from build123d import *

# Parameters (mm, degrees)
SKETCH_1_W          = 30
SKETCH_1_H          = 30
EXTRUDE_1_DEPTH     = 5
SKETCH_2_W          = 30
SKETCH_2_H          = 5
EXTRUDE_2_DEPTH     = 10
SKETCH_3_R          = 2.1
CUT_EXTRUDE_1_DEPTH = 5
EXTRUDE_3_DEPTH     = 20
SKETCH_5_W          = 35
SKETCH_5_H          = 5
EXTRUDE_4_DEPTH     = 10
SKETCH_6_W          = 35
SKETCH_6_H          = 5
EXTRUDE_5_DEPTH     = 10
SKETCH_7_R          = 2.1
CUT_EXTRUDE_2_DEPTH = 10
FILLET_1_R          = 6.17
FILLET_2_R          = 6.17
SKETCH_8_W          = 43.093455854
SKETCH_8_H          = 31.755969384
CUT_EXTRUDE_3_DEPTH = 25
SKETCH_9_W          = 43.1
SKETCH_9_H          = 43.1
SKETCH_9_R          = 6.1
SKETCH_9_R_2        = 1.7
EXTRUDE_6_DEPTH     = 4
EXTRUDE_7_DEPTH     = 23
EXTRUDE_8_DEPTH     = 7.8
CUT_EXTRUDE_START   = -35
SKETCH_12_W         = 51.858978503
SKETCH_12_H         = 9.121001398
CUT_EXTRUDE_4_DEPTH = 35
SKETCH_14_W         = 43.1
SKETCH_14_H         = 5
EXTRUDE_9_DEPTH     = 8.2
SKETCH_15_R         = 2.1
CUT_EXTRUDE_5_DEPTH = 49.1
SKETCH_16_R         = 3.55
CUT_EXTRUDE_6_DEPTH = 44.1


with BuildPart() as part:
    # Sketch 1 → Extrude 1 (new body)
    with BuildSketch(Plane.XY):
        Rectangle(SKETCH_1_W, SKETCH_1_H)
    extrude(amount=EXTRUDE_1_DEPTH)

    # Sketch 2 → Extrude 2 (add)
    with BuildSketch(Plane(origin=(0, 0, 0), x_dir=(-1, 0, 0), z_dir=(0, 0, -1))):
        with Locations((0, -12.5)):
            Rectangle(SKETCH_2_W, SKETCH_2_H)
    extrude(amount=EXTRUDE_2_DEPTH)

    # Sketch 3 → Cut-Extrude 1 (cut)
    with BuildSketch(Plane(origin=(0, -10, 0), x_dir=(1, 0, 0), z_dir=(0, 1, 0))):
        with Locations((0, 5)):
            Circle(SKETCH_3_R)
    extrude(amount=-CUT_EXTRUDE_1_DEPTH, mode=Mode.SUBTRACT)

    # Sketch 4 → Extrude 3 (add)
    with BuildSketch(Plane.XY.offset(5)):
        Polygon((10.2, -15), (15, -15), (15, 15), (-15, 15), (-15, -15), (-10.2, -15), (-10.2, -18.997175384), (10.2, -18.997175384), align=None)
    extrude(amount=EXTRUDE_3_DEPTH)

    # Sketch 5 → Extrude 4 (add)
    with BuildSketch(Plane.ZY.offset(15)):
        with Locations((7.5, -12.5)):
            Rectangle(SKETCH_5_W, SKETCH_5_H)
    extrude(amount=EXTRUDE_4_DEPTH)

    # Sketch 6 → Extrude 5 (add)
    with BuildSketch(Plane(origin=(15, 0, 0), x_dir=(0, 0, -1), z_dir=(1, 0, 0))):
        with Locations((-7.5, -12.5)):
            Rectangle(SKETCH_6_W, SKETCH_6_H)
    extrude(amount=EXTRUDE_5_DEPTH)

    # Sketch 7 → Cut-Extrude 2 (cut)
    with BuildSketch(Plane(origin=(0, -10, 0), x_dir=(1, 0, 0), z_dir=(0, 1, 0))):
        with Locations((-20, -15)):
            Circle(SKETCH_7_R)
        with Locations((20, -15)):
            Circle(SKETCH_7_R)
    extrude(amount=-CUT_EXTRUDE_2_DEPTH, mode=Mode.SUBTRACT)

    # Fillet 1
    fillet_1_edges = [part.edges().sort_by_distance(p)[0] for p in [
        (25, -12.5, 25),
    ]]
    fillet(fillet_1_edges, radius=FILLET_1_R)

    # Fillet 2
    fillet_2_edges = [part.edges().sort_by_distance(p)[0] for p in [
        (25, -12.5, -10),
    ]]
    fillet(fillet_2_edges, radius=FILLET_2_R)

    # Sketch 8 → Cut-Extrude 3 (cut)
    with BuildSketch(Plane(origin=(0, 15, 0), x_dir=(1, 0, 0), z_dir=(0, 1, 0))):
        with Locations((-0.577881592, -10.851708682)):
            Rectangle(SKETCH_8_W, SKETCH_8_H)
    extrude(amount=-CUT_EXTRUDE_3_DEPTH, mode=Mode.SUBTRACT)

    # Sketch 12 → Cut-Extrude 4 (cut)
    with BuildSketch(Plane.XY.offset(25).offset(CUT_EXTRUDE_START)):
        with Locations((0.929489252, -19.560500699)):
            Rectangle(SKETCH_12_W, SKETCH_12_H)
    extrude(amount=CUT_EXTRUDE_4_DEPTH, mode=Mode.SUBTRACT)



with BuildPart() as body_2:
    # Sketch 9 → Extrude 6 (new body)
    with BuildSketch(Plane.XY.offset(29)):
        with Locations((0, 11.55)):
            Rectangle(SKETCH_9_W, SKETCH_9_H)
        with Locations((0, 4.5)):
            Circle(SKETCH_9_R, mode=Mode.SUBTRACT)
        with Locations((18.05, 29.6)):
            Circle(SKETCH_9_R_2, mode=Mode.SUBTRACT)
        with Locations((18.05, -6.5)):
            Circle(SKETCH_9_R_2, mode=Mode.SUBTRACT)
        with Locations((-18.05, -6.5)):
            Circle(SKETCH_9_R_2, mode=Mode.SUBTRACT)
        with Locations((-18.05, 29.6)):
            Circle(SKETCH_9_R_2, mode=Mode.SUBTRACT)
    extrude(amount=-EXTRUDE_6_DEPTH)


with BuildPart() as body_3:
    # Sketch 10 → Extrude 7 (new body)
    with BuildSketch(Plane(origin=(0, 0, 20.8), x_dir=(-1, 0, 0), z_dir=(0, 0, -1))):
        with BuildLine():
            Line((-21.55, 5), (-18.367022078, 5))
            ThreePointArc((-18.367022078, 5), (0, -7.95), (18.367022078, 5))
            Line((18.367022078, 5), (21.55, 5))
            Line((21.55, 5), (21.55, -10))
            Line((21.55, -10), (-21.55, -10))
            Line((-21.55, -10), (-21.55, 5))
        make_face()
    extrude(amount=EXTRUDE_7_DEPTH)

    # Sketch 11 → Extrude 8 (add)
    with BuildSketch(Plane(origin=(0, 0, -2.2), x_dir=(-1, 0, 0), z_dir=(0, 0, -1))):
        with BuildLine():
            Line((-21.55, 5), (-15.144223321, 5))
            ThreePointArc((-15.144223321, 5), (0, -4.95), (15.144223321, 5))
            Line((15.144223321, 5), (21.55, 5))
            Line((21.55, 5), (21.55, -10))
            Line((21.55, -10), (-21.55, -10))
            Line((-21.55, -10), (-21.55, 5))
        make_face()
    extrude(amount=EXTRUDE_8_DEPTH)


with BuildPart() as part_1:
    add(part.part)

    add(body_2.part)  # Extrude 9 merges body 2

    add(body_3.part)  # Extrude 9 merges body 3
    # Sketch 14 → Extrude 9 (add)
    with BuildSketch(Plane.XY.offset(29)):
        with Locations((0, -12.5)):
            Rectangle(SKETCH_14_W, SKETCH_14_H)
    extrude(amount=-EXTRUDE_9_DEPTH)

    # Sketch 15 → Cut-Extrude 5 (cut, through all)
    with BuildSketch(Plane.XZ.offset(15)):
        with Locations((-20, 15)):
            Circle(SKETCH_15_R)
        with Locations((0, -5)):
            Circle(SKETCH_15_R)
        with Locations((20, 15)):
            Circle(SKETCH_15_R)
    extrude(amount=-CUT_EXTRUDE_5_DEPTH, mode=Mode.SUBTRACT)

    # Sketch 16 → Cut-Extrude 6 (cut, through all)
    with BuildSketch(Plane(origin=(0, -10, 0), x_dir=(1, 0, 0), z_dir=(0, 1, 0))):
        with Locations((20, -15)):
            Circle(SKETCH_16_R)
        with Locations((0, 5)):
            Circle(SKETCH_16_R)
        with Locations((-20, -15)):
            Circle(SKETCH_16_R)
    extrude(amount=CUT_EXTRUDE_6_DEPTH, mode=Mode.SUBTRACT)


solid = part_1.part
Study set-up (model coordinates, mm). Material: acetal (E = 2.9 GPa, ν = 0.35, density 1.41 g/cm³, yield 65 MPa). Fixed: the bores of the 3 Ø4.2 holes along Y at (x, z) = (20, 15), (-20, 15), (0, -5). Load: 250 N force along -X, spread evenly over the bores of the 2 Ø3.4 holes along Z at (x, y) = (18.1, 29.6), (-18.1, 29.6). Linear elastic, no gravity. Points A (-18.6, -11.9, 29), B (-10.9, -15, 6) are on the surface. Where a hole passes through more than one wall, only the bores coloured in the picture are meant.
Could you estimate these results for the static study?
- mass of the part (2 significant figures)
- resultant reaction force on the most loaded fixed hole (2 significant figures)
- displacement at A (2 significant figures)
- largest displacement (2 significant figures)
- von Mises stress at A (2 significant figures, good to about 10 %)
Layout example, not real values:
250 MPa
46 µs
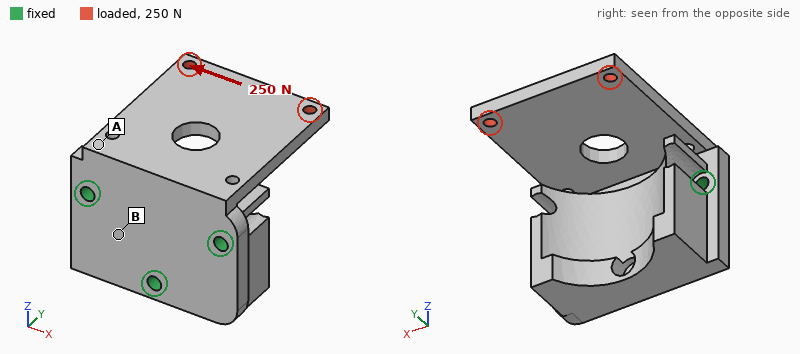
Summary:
36 g
320 N
0.23 mm
0.82 mm
7.1 MPa
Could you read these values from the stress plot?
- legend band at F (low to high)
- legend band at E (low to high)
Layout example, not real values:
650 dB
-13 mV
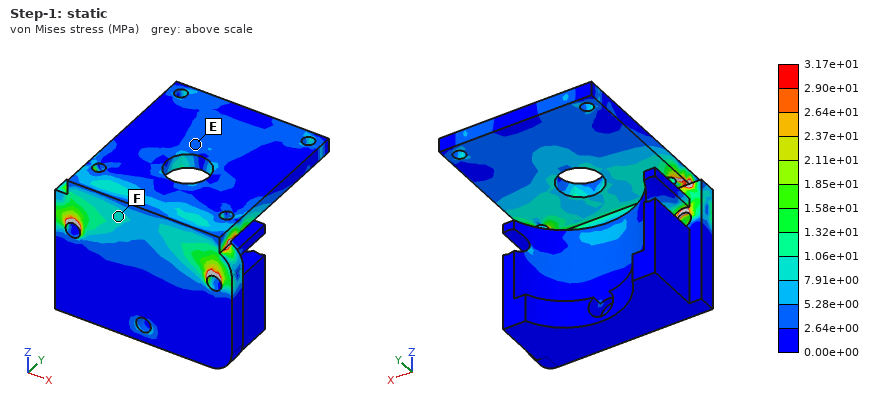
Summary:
7.91e+00 to 1.06e+01 MPa
2.64e+00 to 5.28e+00 MPa
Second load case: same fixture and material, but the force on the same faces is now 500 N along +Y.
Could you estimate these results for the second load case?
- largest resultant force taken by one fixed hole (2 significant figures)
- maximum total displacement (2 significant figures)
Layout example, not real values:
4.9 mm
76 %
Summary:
330 N
0.94 mm
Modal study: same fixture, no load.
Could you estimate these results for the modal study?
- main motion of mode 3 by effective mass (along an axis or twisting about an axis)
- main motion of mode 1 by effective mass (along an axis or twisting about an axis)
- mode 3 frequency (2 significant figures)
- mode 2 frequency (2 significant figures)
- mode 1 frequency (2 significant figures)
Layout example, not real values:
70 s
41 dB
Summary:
along X
along Z
1500 Hz
1000 Hz
380 Hz
